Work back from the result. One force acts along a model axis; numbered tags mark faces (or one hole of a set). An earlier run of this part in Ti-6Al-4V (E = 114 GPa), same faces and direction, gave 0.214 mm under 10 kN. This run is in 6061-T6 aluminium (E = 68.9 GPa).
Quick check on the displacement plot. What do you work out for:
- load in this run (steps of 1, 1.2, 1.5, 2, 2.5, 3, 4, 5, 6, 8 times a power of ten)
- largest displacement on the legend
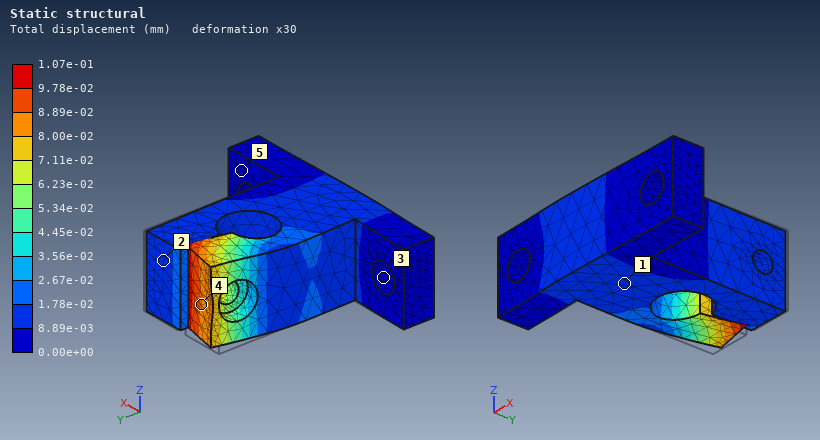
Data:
3 kN
1.07e-01 mm
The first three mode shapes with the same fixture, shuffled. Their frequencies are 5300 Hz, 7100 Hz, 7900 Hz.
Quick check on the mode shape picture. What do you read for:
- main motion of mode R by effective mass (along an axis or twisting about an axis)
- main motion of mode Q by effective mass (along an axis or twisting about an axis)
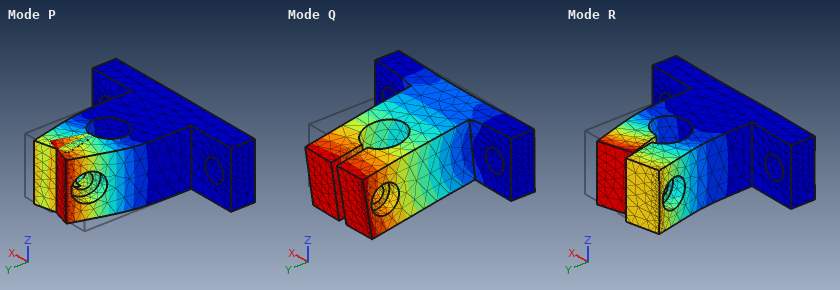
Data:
along X
along Z
